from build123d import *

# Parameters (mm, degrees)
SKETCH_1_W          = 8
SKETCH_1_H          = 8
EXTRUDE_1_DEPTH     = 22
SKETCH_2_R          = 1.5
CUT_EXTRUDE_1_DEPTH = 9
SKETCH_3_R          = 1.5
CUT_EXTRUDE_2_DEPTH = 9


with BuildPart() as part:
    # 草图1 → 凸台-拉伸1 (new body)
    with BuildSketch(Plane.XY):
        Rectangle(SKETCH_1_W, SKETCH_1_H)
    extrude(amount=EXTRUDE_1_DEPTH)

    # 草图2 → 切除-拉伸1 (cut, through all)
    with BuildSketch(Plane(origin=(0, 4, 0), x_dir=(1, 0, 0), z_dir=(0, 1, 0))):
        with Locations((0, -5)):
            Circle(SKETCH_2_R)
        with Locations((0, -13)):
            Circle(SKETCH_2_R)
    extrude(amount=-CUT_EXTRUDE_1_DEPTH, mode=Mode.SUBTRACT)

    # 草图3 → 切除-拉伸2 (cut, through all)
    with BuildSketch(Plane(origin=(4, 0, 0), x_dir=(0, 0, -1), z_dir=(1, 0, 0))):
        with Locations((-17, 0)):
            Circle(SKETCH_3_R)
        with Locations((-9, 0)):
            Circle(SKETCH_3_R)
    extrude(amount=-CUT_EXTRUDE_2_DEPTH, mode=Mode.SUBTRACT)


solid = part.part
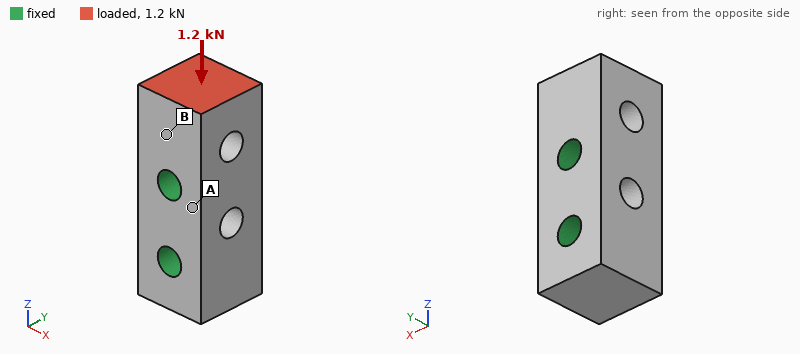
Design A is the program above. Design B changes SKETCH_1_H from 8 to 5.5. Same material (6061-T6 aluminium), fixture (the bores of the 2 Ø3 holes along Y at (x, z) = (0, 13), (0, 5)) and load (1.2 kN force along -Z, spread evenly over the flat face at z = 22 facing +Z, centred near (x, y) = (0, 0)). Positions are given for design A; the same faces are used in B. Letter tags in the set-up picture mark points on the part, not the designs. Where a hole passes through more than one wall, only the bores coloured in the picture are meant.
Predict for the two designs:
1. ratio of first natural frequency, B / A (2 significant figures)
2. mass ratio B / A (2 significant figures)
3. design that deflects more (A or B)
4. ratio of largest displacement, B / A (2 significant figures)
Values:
0.86
0.66
B
1.7
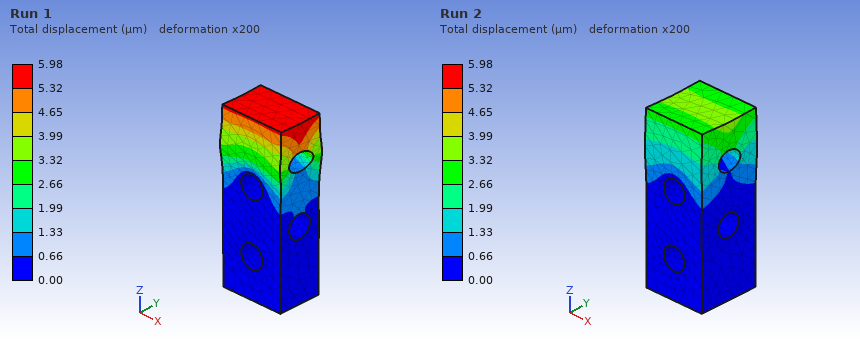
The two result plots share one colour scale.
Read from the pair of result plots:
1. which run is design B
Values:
Run 1
